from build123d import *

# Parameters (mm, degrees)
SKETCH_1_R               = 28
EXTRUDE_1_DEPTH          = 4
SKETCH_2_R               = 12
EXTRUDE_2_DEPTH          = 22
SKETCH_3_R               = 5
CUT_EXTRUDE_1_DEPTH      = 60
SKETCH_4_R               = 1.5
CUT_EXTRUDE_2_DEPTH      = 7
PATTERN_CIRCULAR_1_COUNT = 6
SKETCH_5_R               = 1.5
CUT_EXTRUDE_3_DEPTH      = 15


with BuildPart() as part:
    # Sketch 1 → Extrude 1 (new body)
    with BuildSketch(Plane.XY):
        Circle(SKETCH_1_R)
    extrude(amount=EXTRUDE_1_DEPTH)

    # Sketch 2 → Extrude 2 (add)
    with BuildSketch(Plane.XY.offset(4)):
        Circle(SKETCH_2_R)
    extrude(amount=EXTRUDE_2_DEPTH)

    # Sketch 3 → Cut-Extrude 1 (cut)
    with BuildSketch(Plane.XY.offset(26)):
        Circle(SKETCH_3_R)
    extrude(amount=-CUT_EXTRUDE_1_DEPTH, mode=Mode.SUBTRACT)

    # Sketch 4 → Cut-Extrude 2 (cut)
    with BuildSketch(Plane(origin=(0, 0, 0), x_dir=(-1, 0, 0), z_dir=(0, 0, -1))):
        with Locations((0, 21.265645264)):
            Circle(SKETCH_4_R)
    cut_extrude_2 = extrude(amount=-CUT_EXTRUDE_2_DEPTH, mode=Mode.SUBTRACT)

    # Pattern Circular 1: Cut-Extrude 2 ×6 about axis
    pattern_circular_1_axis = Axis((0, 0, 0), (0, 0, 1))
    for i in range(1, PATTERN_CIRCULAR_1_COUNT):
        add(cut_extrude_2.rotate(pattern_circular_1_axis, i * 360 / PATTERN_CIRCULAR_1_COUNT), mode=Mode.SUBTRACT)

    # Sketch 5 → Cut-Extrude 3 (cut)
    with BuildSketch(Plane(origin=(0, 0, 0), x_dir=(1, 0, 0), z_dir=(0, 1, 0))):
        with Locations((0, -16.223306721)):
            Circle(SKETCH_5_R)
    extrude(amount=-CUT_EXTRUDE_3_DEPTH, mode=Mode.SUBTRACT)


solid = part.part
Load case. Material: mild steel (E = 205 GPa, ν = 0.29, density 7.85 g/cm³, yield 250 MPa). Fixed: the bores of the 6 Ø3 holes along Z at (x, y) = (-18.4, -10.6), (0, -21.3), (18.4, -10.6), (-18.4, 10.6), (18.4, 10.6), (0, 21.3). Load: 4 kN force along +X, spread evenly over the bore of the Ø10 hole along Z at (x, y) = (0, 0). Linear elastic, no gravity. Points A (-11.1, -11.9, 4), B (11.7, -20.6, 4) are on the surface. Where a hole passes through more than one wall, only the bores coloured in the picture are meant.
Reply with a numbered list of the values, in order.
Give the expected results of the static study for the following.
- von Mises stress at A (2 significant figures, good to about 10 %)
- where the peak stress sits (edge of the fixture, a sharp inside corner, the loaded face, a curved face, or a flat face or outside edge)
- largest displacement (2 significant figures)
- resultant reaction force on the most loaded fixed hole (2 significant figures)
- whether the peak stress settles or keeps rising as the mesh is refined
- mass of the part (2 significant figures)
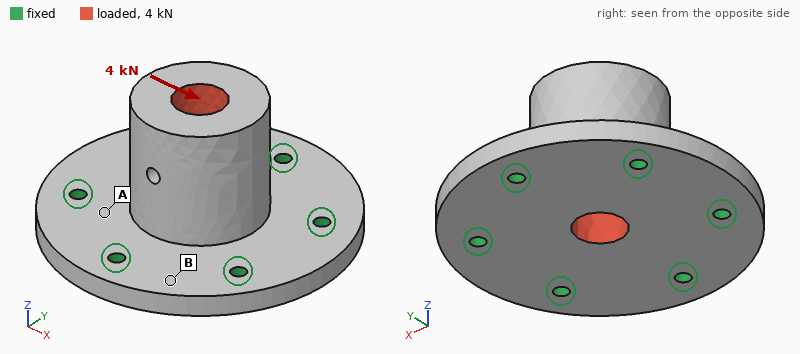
1. 36 MPa
2. edge of the fixture
3. 18 µm
4. 1.1 kN
5. keeps rising
6. 140 g
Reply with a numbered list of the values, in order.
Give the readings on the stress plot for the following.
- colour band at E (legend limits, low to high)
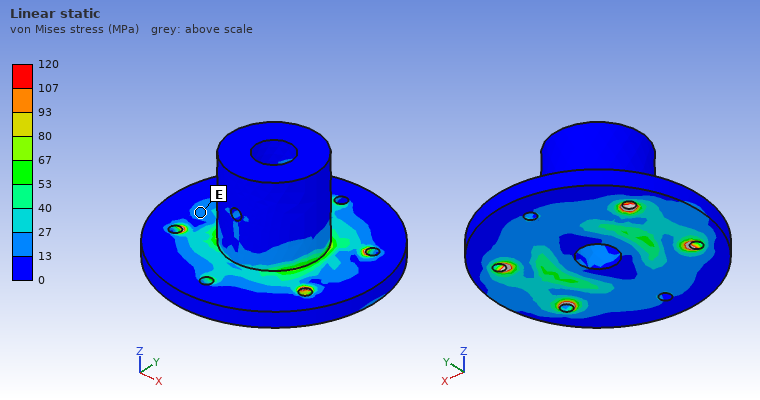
1. 13 to 27 MPa
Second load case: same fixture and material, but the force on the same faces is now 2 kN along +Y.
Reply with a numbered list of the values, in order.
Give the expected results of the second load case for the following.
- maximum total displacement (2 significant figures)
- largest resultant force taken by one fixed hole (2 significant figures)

1. 8.9 µm
2. 640 N
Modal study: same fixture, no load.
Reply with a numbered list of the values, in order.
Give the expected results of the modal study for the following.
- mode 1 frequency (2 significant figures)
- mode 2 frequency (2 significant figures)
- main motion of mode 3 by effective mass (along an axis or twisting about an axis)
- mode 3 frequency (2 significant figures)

1. 10000 Hz
2. 10 kHz
3. along Z
4. 13 kHz
